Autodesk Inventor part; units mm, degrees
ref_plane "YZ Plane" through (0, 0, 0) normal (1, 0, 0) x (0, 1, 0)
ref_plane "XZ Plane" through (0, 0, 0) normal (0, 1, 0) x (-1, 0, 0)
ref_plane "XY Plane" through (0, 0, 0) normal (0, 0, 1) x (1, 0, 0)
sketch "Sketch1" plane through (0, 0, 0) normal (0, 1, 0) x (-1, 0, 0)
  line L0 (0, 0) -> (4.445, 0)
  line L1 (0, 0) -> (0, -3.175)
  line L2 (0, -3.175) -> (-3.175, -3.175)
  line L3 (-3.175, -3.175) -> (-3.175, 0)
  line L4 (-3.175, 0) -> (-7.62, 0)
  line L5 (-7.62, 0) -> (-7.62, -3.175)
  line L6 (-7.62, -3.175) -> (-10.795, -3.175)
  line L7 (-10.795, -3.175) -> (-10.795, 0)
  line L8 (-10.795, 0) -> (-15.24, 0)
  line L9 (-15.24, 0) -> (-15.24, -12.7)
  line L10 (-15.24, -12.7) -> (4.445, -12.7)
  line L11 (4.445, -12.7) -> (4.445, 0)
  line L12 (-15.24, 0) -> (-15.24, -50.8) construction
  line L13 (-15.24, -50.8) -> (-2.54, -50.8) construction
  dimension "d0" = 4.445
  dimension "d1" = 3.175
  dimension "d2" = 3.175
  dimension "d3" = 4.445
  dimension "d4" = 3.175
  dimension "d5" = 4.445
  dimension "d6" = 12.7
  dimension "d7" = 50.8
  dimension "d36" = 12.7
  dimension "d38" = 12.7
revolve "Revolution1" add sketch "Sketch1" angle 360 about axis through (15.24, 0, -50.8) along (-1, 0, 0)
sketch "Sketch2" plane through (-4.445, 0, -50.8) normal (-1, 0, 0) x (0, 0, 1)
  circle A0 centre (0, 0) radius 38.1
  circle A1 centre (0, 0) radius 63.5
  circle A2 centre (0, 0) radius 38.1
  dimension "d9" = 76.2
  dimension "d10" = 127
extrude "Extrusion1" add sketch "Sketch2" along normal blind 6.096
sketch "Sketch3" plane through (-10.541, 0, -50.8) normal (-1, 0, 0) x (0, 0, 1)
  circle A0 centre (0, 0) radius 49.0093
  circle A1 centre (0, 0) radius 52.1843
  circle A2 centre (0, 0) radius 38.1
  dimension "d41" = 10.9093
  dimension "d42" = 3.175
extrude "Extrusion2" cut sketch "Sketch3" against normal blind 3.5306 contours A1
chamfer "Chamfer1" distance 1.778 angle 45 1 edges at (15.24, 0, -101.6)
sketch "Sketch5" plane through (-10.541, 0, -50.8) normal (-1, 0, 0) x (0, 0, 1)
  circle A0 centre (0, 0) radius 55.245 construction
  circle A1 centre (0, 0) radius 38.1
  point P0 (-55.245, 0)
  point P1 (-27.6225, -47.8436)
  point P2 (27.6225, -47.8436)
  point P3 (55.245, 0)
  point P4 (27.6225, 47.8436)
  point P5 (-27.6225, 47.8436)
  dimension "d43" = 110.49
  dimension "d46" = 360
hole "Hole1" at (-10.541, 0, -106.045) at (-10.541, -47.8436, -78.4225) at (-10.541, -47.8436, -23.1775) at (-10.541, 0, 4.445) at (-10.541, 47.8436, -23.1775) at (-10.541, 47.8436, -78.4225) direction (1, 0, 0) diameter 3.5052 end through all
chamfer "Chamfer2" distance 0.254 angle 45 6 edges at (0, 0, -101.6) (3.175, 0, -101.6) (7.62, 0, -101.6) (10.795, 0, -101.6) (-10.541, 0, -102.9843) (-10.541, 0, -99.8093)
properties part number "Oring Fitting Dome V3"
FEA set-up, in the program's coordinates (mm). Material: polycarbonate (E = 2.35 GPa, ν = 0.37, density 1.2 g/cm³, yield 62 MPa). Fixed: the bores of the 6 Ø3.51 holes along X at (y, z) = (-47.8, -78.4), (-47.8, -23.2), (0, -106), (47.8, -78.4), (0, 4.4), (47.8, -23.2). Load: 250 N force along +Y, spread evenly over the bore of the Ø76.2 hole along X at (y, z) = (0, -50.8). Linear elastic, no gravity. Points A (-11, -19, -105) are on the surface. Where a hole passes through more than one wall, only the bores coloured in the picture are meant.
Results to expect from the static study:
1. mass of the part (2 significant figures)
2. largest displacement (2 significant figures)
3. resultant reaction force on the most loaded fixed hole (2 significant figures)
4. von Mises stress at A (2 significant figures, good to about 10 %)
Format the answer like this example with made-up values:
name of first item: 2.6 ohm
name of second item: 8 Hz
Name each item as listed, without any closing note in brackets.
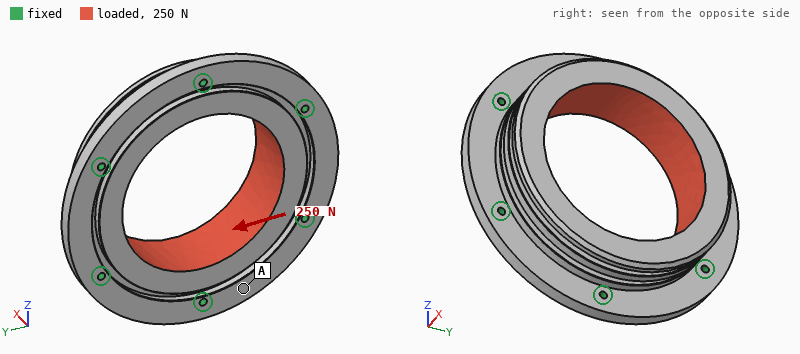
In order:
mass of the part: 130 g
largest displacement: 8.7 µm
resultant reaction force on the most loaded fixed hole: 44 N
von Mises stress at A: 0.13 MPa
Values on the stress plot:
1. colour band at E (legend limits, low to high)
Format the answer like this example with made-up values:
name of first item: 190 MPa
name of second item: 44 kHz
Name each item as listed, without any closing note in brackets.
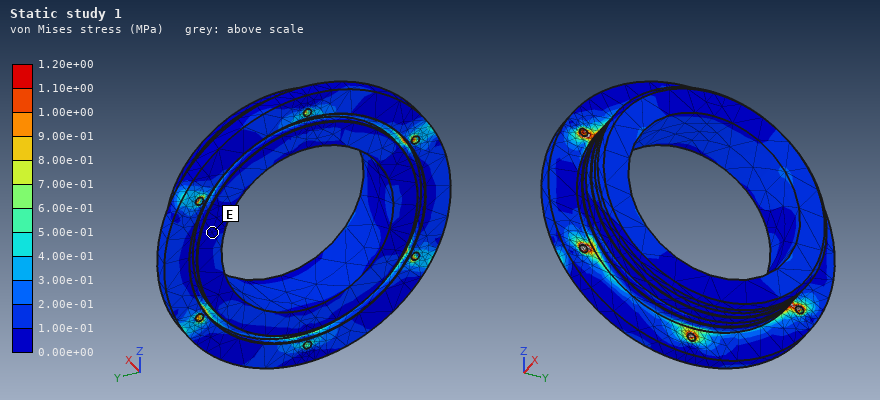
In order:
colour band at E: 0.00e+00 to 1.00e-01 MPa
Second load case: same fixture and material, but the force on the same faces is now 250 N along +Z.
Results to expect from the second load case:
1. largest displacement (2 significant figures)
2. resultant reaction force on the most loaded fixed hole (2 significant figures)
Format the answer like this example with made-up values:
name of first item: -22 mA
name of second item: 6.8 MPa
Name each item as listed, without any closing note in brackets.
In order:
largest displacement: 8.1 µm
resultant reaction force on the most loaded fixed hole: 45 N
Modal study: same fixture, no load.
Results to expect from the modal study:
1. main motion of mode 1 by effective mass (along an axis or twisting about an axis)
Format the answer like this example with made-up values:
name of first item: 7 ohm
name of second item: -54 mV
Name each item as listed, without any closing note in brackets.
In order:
main motion of mode 1 by effective mass: along X
